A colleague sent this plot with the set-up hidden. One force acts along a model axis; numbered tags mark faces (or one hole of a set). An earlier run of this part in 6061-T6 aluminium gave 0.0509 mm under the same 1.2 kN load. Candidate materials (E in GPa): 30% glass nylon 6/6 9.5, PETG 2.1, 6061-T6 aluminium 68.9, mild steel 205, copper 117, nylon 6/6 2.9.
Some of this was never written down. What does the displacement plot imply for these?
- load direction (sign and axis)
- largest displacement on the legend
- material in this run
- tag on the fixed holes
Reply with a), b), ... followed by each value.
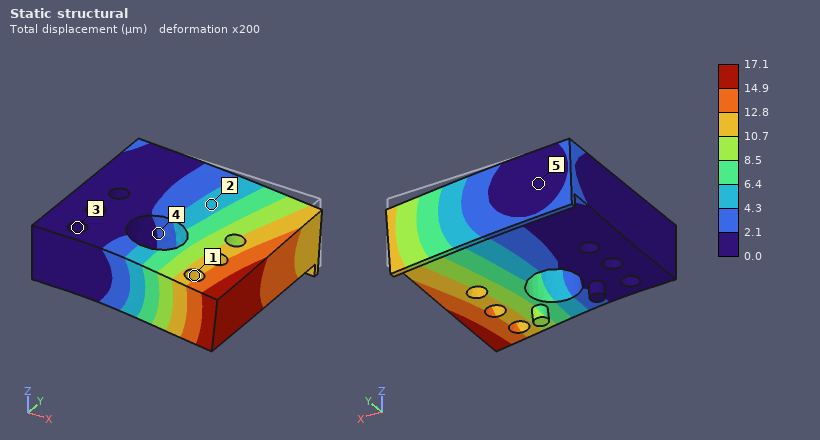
a) -Z
b) 17.1 µm
c) mild steel
d) 3
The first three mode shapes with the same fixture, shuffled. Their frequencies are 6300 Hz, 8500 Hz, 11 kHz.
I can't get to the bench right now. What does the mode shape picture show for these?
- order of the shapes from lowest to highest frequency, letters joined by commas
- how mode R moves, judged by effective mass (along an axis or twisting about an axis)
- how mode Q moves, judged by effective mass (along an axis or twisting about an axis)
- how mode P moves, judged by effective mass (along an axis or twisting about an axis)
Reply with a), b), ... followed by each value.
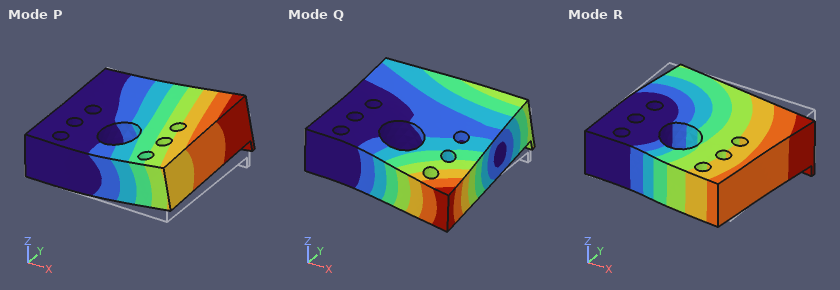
a) P, R, Q
b) along Y
c) twisting about X
d) along Z
